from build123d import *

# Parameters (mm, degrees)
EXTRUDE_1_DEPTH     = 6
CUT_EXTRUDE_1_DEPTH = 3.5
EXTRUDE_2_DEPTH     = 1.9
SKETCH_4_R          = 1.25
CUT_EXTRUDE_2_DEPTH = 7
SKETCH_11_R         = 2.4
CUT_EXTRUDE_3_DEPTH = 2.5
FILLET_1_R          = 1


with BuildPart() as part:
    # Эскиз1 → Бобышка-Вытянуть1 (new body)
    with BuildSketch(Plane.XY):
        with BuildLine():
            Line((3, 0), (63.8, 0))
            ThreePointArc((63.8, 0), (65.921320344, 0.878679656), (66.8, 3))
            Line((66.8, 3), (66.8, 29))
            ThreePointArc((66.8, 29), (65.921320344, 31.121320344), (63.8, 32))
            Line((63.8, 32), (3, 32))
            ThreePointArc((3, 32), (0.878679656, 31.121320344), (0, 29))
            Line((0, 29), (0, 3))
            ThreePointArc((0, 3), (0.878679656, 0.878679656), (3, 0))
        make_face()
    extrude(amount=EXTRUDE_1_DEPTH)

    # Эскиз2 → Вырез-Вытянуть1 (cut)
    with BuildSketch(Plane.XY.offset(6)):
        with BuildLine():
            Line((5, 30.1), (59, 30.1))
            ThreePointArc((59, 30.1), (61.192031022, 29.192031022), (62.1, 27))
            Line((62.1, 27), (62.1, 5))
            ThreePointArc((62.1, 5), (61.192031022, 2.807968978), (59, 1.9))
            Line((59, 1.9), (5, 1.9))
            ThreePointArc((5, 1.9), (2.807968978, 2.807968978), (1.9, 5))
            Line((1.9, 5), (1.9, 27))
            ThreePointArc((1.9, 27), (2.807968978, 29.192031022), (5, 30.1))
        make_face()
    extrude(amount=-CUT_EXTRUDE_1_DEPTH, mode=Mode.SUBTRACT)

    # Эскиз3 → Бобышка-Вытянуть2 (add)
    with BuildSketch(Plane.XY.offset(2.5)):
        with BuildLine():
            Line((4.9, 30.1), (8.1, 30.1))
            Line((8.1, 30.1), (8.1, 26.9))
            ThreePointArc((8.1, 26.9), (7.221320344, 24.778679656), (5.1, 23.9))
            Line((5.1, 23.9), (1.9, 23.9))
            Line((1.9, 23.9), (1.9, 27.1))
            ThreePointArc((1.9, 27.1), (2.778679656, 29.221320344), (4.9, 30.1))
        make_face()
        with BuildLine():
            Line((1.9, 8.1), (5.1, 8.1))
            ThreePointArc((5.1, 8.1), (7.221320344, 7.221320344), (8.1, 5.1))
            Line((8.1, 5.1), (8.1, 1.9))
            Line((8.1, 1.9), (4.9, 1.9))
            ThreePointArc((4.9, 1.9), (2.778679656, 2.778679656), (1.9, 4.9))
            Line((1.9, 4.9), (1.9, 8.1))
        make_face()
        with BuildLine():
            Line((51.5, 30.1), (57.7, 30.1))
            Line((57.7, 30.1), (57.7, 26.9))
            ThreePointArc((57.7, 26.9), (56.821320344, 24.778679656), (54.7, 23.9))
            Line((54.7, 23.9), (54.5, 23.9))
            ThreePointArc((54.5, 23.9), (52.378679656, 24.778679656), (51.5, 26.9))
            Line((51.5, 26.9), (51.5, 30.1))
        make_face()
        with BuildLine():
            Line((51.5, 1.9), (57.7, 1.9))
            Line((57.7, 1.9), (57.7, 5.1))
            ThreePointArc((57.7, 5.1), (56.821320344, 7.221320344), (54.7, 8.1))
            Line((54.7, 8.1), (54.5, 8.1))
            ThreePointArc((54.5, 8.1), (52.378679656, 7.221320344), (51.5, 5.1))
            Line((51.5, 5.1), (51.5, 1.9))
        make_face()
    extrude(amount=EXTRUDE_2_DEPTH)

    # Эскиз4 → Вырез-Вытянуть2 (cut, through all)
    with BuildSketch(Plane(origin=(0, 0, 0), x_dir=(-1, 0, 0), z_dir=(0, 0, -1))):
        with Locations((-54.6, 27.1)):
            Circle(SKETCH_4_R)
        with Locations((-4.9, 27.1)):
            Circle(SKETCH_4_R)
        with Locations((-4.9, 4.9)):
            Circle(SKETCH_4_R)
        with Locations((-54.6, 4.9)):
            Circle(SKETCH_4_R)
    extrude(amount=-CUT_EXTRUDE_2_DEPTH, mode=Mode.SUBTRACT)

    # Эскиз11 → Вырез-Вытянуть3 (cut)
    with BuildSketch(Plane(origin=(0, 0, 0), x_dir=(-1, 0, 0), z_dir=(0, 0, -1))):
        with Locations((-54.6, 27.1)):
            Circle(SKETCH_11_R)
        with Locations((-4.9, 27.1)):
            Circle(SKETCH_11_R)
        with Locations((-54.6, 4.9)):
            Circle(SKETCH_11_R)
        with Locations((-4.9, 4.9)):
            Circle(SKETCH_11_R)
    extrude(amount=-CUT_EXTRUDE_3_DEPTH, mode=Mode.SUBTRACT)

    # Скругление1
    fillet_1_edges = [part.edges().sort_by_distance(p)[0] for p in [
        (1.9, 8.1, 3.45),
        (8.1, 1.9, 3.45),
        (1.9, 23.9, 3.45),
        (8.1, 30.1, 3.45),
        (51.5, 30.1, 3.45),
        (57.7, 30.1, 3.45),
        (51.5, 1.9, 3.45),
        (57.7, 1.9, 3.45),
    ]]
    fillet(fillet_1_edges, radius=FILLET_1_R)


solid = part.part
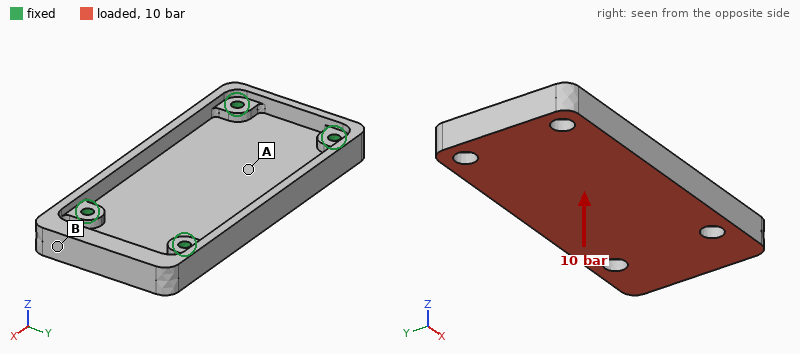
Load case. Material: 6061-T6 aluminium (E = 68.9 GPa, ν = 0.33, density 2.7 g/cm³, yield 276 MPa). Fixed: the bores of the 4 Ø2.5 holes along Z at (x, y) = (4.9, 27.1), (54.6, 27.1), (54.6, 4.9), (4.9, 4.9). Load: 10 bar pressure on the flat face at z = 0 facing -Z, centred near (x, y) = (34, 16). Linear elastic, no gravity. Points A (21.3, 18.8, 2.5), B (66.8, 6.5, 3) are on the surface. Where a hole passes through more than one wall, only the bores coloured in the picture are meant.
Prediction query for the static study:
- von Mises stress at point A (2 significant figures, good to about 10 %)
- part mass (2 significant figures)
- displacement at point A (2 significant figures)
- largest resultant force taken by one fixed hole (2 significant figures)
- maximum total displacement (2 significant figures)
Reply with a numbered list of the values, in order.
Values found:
1. 37 MPa
2. 19 g
3. 0.093 mm
4. 750 N
5. 0.11 mm
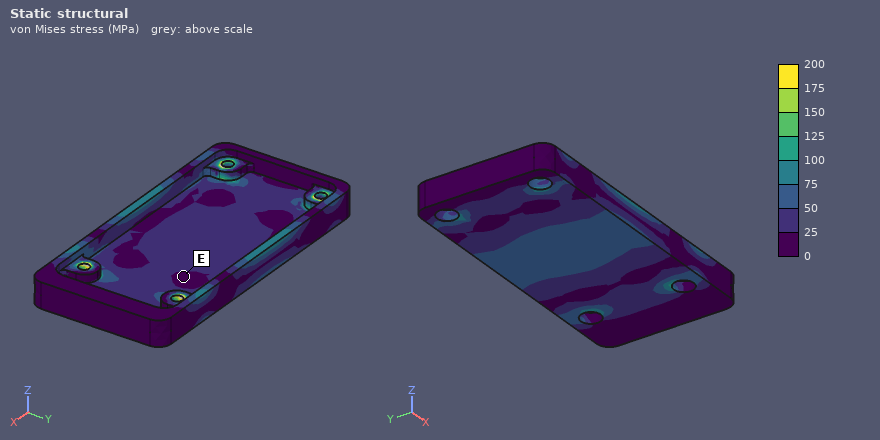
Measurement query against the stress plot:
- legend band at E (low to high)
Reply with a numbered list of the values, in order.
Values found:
1. 0 to 25 MPa
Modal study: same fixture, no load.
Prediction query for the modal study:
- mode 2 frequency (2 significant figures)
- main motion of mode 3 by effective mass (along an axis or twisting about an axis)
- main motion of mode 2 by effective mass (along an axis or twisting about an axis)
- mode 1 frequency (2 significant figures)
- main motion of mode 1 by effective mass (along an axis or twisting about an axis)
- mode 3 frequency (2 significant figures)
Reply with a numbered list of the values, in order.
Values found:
1. 8800 Hz
2. along Z
3. twisting about X
4. 6100 Hz
5. along Z
6. 10 kHz
